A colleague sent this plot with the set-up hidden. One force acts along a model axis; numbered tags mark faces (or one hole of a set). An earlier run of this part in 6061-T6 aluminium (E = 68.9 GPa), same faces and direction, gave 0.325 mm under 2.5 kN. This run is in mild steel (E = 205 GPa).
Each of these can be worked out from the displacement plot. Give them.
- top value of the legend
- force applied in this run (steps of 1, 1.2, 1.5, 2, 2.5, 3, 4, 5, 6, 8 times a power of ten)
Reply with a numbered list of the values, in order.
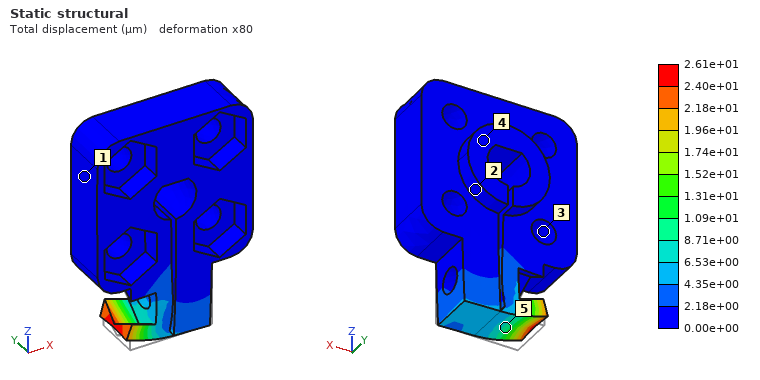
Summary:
1. 2.61e+01 µm
2. 600 N
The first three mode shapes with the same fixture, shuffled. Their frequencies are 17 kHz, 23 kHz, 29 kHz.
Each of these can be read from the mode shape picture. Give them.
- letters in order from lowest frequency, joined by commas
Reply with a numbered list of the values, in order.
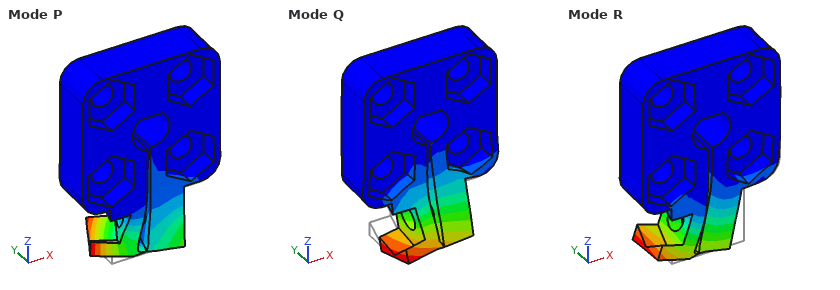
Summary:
1. Q, R, P
